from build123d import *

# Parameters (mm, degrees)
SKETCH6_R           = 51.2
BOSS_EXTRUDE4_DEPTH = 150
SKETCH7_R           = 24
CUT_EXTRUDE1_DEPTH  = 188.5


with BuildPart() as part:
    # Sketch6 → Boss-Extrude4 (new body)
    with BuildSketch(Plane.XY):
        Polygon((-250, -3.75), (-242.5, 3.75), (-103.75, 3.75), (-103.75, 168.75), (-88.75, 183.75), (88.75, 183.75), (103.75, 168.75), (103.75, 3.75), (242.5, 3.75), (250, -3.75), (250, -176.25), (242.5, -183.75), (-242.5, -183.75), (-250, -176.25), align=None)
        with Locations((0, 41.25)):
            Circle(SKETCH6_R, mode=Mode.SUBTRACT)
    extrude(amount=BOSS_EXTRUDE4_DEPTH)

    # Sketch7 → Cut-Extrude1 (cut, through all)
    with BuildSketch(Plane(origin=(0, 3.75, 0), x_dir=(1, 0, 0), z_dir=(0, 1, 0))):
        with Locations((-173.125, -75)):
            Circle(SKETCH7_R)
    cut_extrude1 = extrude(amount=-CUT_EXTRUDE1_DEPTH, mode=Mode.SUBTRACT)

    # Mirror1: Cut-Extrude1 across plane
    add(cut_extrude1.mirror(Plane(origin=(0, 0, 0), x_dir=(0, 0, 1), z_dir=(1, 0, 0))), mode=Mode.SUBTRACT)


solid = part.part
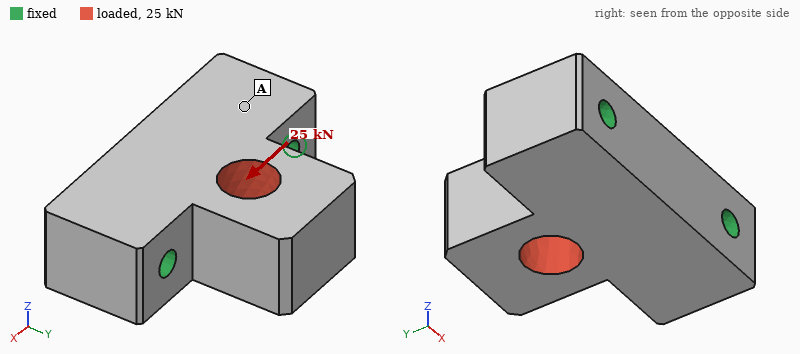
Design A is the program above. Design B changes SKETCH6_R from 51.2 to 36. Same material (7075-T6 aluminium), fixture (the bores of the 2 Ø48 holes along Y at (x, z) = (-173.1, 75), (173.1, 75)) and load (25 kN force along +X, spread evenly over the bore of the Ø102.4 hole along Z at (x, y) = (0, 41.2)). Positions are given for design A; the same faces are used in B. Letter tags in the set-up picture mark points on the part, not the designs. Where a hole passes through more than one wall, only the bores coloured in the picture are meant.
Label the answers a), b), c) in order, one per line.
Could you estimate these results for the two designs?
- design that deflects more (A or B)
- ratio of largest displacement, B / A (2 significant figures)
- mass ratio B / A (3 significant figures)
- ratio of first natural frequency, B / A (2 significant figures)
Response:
a) A
b) 0.73
c) 1.04
d) 1.0
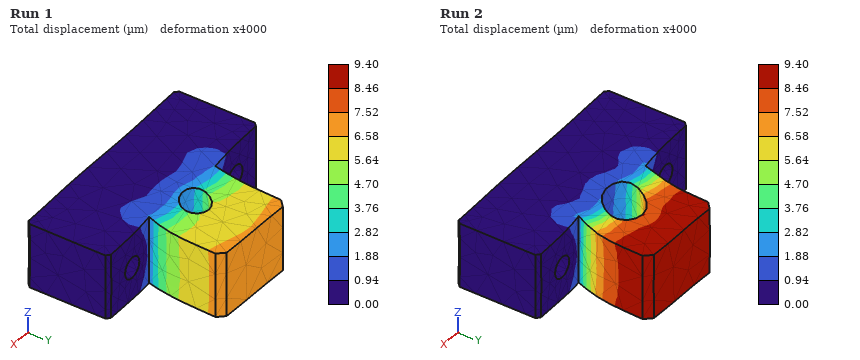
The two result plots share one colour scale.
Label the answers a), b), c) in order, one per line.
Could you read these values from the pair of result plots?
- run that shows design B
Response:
a) Run 1
